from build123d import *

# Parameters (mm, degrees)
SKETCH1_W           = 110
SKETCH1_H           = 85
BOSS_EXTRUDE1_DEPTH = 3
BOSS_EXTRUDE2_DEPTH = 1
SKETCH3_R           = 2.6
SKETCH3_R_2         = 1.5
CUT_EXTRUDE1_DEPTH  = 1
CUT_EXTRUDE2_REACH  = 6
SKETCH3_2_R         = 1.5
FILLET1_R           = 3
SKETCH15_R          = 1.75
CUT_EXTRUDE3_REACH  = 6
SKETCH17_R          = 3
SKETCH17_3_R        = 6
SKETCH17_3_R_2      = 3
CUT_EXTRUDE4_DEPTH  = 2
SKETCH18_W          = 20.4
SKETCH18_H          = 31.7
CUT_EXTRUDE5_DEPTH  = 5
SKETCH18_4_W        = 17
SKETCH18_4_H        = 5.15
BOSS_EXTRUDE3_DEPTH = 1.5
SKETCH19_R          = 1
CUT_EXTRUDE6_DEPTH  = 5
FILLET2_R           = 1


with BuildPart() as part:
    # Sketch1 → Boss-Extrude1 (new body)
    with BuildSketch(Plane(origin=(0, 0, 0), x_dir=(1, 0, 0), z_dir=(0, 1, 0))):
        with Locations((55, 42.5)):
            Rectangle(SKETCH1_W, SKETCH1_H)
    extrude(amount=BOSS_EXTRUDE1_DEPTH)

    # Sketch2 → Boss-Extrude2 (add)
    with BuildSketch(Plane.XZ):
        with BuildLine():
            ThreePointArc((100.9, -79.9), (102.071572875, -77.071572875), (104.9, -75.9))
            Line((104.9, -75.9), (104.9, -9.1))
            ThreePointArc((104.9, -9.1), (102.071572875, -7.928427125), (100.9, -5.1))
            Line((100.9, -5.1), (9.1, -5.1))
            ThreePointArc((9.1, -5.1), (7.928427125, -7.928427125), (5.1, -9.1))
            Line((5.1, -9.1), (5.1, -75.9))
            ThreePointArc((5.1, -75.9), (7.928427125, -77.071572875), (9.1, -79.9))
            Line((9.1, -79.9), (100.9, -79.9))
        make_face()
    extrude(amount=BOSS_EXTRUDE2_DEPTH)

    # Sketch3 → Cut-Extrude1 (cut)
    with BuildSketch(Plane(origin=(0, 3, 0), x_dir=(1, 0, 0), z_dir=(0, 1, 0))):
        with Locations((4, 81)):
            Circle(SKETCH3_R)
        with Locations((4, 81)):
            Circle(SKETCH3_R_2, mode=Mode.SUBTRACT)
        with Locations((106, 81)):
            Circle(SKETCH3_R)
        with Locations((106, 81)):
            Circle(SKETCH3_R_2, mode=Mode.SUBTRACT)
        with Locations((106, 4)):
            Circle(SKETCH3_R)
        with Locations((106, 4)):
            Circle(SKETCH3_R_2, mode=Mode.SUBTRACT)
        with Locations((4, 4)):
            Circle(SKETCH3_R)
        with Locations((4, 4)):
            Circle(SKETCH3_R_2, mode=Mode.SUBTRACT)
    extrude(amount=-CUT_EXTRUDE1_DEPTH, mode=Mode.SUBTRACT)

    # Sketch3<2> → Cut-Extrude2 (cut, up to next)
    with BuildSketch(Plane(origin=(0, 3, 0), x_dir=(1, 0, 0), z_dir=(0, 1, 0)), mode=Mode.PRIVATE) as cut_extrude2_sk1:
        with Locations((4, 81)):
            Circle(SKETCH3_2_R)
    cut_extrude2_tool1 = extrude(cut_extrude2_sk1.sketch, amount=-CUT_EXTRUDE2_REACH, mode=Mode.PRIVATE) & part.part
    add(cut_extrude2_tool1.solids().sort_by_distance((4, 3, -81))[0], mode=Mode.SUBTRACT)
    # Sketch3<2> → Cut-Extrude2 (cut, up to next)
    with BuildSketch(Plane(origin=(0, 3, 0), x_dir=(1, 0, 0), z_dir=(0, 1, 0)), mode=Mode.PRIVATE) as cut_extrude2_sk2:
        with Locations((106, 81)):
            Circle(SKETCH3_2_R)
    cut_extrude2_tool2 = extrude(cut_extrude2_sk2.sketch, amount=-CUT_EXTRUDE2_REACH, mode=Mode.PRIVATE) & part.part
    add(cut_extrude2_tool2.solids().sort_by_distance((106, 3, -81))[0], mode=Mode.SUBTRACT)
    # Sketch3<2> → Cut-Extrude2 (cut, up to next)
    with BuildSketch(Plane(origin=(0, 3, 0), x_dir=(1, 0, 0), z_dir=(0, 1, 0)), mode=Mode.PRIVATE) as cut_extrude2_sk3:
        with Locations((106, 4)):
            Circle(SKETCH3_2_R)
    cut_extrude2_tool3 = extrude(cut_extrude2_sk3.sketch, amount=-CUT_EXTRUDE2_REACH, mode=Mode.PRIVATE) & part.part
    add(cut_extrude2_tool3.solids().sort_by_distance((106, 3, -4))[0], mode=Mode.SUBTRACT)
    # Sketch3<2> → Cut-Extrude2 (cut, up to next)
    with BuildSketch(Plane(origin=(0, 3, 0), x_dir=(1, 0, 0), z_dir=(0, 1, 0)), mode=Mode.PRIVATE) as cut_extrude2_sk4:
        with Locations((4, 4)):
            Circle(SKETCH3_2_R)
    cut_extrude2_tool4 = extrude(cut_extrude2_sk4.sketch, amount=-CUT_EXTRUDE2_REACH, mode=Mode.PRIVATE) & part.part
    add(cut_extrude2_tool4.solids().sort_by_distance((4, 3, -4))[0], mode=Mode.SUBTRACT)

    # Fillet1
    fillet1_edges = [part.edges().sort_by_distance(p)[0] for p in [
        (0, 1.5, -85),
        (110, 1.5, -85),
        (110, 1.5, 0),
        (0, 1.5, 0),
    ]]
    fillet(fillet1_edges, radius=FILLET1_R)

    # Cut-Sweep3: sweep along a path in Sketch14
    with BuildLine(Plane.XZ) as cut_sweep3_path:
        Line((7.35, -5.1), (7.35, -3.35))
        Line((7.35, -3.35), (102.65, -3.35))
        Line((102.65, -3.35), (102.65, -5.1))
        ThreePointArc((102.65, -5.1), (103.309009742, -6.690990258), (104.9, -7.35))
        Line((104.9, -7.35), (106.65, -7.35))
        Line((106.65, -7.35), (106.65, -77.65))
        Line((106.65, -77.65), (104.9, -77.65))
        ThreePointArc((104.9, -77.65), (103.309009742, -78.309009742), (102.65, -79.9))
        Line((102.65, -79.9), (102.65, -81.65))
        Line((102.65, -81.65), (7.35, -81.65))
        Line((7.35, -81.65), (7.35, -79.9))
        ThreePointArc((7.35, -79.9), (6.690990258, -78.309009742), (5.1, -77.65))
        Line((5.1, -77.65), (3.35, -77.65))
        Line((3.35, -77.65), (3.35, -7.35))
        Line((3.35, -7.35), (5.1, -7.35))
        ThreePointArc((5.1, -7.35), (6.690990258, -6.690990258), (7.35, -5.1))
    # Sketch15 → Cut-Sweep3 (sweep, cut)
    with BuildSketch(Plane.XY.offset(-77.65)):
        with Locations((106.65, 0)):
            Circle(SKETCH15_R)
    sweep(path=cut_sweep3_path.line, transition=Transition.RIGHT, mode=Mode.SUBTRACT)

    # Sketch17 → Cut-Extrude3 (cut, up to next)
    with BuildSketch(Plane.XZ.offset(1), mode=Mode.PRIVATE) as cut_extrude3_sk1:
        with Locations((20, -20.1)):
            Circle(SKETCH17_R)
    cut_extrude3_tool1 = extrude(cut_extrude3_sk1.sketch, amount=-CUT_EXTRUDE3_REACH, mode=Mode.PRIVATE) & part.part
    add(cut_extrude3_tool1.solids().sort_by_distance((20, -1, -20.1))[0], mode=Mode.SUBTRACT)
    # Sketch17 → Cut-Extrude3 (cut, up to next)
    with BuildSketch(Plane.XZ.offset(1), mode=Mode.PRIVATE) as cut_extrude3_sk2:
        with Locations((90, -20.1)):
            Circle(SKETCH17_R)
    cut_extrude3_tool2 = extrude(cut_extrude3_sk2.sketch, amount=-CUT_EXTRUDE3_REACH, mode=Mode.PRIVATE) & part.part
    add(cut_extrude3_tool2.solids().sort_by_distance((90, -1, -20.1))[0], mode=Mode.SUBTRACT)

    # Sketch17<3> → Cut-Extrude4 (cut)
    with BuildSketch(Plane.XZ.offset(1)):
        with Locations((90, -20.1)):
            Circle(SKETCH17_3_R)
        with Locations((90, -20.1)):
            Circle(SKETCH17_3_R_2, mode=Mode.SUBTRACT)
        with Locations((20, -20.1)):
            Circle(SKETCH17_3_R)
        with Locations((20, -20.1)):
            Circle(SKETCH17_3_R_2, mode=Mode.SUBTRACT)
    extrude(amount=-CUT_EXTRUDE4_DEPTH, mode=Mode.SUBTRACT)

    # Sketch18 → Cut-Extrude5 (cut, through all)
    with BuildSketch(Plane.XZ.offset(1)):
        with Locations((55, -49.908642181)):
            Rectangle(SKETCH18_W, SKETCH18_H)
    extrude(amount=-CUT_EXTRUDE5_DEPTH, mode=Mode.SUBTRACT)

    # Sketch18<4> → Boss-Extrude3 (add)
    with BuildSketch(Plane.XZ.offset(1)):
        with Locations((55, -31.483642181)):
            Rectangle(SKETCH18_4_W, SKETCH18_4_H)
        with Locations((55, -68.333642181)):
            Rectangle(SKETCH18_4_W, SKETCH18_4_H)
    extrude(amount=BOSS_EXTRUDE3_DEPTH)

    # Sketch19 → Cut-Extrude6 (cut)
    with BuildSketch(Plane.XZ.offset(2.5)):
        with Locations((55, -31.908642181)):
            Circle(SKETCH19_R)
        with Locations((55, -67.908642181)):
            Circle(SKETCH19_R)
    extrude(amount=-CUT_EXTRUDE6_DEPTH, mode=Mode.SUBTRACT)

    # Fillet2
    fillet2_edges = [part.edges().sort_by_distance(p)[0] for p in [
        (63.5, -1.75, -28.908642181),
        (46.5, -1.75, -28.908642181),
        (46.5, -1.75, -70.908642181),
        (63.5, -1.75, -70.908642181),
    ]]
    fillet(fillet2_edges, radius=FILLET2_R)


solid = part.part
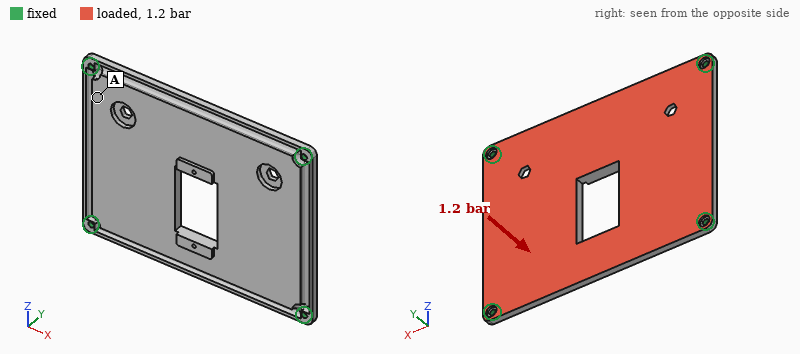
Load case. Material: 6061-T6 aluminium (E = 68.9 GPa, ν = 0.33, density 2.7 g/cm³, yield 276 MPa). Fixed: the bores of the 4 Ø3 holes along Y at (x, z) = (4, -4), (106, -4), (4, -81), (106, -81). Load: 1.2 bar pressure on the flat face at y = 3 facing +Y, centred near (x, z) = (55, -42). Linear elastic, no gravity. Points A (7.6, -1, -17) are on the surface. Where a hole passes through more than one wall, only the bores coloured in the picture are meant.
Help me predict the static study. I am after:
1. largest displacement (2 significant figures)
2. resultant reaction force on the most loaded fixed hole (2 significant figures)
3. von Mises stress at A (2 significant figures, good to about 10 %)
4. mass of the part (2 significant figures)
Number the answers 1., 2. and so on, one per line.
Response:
1. 0.45 mm
2. 510 N
3. 33 MPa
4. 83 g
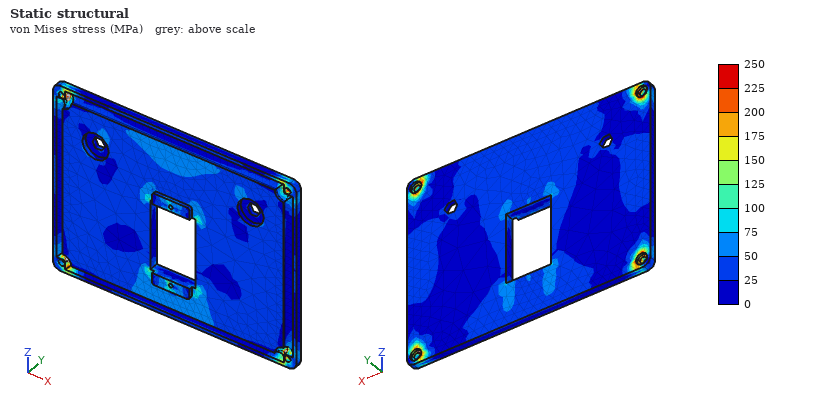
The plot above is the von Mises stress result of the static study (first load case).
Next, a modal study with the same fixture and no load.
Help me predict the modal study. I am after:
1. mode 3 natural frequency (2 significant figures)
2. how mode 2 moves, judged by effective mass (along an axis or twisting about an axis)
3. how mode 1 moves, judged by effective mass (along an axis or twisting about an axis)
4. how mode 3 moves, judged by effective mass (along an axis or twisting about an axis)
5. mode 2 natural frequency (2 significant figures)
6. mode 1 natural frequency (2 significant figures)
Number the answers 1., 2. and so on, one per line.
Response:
1. 2200 Hz
2. twisting about X
3. along Y
4. twisting about Z
5. 1900 Hz
6. 960 Hz
